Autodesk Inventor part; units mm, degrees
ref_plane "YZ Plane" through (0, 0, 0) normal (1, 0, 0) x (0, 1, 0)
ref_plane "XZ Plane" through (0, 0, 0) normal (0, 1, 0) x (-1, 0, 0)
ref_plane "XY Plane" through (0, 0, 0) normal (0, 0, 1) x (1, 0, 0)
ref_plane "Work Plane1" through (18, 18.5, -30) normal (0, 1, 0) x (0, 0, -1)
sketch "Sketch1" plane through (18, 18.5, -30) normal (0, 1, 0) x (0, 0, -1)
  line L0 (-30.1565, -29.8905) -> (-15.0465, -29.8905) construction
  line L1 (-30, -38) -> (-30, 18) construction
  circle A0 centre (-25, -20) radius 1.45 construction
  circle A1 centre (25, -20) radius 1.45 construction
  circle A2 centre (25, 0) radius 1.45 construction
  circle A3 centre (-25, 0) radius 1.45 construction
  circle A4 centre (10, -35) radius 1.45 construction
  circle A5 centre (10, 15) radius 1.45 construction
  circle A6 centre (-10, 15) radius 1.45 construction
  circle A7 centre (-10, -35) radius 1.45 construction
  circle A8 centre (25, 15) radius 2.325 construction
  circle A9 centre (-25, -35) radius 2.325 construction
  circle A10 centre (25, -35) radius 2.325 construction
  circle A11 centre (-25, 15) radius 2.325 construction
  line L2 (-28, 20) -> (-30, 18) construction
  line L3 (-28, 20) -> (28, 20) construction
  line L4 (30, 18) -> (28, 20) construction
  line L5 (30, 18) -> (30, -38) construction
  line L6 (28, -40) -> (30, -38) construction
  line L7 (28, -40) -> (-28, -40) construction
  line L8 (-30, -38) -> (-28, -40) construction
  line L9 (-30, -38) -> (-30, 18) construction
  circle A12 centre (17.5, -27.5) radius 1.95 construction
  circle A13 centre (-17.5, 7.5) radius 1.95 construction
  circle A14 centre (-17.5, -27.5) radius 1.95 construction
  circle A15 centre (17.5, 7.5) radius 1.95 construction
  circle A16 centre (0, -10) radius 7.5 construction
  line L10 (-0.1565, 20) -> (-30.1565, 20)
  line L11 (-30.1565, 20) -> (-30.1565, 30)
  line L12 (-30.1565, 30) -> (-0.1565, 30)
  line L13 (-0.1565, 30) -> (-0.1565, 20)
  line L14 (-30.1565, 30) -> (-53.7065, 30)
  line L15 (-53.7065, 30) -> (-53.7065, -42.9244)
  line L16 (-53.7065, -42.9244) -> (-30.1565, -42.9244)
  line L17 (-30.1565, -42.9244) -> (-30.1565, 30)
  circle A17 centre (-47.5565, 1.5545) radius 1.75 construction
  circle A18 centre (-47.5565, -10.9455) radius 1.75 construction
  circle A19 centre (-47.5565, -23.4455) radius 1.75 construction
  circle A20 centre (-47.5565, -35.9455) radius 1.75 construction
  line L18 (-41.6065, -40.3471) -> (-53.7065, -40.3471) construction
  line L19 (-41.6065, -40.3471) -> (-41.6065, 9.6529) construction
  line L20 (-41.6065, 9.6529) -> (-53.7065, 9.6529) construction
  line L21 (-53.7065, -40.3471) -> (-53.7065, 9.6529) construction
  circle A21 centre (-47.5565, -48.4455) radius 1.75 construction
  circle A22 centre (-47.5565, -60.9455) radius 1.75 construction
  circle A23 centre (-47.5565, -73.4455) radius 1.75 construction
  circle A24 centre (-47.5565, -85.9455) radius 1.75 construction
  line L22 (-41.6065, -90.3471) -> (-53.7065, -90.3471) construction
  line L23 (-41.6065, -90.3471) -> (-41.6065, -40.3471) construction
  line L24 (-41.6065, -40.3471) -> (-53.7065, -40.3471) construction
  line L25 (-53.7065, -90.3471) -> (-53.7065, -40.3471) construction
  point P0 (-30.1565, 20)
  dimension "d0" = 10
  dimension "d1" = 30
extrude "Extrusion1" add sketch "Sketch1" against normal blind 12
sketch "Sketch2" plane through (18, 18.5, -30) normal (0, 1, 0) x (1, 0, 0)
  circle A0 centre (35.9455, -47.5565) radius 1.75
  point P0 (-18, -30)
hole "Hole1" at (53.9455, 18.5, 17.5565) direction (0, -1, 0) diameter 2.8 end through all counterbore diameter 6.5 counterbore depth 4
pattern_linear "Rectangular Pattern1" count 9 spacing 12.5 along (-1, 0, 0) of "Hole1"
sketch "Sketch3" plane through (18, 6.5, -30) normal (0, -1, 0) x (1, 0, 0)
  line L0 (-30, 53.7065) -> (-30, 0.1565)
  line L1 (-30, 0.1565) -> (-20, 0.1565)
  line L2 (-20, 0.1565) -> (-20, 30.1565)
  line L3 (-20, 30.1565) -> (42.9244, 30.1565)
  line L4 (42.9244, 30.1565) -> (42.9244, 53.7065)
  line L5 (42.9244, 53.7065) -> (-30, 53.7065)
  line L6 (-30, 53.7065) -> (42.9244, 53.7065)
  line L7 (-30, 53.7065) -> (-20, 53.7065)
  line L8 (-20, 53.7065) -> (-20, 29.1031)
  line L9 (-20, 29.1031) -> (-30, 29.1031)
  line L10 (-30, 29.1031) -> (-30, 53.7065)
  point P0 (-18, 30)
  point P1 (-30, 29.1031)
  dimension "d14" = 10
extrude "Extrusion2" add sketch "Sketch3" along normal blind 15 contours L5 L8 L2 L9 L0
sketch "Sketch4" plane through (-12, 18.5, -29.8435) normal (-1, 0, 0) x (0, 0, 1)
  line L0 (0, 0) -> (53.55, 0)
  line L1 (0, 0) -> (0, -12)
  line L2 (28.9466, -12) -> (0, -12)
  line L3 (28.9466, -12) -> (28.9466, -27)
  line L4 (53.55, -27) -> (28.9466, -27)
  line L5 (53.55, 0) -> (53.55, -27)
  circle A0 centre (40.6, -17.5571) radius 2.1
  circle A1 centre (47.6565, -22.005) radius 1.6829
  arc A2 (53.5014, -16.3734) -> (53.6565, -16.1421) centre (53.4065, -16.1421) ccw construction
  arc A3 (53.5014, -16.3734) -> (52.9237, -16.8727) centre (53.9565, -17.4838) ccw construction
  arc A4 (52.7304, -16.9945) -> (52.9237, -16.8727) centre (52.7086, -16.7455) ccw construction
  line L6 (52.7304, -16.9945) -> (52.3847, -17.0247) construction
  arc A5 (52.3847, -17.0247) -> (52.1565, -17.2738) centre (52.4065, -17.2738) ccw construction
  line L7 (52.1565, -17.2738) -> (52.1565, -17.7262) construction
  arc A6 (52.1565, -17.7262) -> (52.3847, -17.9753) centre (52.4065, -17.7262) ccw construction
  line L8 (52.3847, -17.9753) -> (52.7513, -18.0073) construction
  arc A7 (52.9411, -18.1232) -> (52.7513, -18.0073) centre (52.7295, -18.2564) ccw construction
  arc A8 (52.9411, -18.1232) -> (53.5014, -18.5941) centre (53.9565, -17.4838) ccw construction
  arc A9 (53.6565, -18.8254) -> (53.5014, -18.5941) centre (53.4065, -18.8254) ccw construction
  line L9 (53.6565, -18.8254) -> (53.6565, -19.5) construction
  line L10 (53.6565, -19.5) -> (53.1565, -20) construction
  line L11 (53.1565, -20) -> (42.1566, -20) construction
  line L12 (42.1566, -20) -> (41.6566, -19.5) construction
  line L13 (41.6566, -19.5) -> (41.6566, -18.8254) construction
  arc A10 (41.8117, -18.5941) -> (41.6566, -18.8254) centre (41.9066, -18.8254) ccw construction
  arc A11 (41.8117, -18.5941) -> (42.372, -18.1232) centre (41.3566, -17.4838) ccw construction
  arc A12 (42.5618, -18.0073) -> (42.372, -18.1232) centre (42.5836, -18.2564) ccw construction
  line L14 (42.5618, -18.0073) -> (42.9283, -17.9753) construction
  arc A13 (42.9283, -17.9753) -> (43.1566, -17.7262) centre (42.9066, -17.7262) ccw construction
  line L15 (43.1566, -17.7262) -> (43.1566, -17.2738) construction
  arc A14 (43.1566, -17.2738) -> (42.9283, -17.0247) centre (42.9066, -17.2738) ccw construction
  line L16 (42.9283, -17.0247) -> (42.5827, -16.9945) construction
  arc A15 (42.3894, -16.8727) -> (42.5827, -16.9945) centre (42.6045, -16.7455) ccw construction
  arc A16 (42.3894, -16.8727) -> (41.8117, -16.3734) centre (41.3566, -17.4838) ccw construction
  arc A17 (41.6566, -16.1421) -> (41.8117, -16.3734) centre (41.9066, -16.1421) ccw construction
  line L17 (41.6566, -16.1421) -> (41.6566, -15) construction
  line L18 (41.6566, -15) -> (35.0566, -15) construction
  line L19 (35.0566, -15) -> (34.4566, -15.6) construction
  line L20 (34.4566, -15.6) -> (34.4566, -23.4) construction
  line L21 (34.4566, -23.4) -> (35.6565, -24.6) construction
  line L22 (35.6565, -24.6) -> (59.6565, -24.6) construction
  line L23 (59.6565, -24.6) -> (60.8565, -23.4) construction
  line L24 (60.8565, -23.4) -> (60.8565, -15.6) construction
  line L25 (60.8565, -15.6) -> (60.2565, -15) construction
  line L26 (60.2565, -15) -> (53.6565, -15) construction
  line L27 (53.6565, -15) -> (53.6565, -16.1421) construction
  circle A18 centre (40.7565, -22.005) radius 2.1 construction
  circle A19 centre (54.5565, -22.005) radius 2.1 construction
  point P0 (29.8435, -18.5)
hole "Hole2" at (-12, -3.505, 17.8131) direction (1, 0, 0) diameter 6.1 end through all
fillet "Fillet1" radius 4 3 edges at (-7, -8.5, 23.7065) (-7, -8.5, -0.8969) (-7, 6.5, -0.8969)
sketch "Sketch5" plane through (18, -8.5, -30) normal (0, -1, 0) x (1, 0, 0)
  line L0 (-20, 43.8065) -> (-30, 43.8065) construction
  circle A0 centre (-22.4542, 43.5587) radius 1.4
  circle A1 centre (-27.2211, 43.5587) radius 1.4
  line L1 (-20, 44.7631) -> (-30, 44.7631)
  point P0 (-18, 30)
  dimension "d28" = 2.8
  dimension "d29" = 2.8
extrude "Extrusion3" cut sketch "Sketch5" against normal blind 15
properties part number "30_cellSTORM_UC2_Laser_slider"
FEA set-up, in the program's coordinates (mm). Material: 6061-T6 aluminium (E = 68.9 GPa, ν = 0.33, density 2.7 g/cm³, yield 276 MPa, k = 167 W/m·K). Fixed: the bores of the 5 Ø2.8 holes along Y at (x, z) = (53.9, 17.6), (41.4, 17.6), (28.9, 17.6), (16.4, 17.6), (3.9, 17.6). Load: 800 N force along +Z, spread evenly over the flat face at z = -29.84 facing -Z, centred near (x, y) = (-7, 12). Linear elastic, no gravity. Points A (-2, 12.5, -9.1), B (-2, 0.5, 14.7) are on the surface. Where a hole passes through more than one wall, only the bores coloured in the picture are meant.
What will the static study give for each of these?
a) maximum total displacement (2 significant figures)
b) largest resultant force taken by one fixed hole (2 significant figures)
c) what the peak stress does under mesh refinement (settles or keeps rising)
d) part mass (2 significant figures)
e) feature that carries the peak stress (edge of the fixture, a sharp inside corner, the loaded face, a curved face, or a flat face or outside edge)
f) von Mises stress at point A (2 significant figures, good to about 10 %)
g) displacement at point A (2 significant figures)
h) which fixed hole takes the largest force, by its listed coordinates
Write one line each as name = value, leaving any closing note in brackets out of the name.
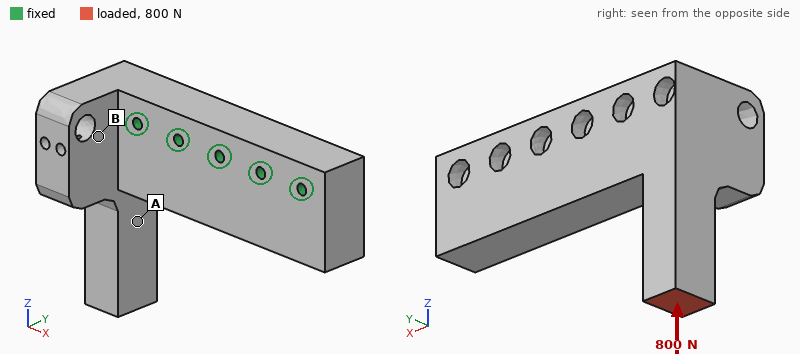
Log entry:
maximum total displacement = 17 µm
largest resultant force taken by one fixed hole = 1.1 kN
what the peak stress does under mesh refinement = keeps rising
part mass = 71 g
feature that carries the peak stress = edge of the fixture
von Mises stress at point A = 6.6 MPa
displacement at point A = 7.8 µm
which fixed hole takes the largest force, by its listed coordinates = (3.9, 17.6)
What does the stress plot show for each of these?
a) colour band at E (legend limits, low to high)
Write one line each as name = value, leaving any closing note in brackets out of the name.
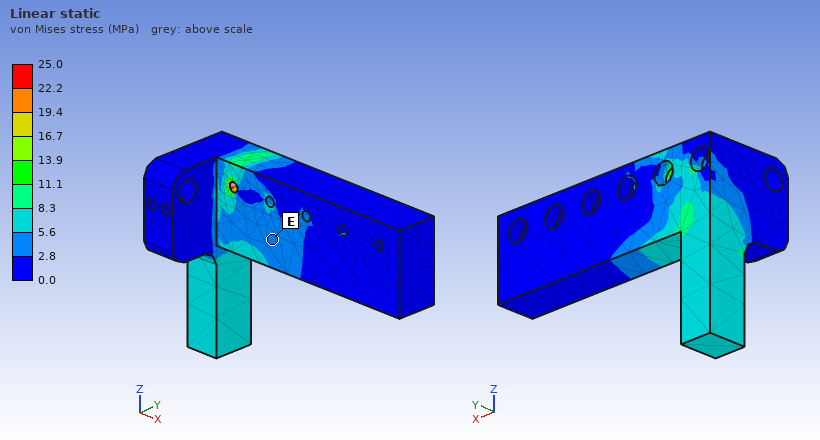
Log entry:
colour band at E = 2.8 to 5.6 MPa
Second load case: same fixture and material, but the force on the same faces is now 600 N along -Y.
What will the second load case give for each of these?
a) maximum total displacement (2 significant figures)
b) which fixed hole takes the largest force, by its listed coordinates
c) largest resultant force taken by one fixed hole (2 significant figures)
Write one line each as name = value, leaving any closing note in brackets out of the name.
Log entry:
maximum total displacement = 0.20 mm
which fixed hole takes the largest force, by its listed coordinates = (3.9, 17.6)
largest resultant force taken by one fixed hole = 570 N
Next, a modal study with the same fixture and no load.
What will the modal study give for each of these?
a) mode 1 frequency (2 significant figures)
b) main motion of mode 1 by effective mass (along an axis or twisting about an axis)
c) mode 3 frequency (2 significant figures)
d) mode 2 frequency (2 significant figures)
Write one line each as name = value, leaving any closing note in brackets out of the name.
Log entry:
mode 1 frequency = 4100 Hz
main motion of mode 1 by effective mass = along Y
mode 3 frequency = 9800 Hz
mode 2 frequency = 5700 Hz
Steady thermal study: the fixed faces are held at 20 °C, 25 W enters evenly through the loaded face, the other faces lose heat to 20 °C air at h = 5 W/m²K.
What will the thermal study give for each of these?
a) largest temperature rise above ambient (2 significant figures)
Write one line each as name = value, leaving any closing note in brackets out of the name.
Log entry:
largest temperature rise above ambient = 51 K
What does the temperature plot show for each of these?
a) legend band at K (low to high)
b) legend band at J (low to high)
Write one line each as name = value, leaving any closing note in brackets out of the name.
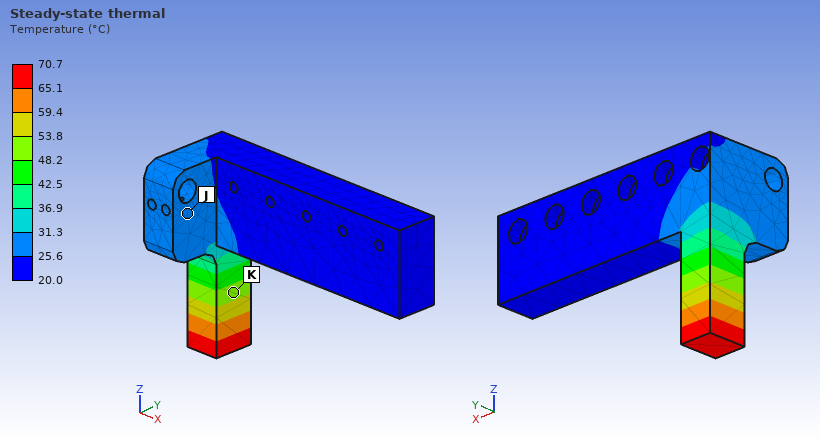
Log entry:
legend band at K = 48.2 to 53.8 °C
legend band at J = 25.6 to 31.3 °C
